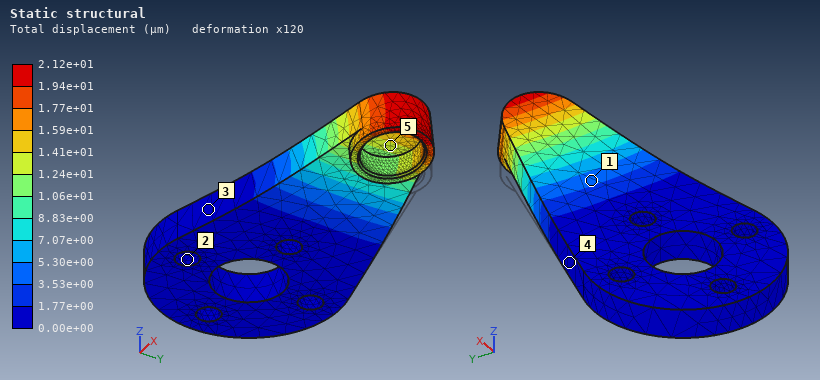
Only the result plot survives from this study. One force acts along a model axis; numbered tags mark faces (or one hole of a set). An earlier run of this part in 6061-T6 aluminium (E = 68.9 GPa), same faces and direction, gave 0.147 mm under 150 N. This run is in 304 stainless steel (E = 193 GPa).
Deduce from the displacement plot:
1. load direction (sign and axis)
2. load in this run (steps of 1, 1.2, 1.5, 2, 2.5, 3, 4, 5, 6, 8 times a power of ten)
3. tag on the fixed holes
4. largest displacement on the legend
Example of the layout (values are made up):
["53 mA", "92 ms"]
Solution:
["+Z", "60 N", "2", "2.12e+01 µm"]
